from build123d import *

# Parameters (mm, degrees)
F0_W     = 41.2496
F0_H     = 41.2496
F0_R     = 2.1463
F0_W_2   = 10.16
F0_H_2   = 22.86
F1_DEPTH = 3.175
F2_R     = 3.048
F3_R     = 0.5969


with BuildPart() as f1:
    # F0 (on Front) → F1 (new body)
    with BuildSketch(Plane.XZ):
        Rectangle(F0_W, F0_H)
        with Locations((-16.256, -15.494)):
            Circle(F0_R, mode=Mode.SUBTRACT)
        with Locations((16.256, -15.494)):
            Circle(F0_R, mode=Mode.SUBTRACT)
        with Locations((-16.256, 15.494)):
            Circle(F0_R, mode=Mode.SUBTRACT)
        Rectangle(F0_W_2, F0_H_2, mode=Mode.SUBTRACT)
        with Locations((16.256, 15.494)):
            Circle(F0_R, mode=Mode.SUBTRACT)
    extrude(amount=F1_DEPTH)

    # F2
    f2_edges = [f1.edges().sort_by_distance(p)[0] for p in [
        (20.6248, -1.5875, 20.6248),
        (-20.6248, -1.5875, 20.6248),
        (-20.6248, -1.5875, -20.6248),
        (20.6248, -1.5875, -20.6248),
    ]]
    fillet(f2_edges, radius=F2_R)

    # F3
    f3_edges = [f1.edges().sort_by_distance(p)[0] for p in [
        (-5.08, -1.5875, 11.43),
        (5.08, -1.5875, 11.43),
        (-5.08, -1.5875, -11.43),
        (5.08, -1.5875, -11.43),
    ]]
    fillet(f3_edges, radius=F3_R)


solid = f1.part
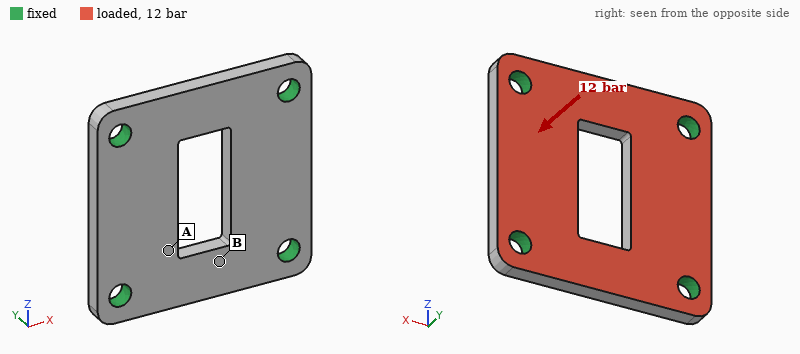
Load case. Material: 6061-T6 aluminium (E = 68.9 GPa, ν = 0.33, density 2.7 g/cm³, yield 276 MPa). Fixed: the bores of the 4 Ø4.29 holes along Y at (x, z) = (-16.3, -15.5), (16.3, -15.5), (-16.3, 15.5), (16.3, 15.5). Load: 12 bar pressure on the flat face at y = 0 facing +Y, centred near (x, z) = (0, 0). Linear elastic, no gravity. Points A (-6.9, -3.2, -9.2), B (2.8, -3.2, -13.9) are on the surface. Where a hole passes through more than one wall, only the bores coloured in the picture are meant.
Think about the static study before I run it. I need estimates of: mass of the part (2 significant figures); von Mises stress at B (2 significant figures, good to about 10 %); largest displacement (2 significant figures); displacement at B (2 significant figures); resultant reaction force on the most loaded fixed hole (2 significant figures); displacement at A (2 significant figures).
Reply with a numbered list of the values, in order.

1. 12 g
2. 28 MPa
3. 33 µm
4. 19 µm
5. 420 N
6. 21 µm
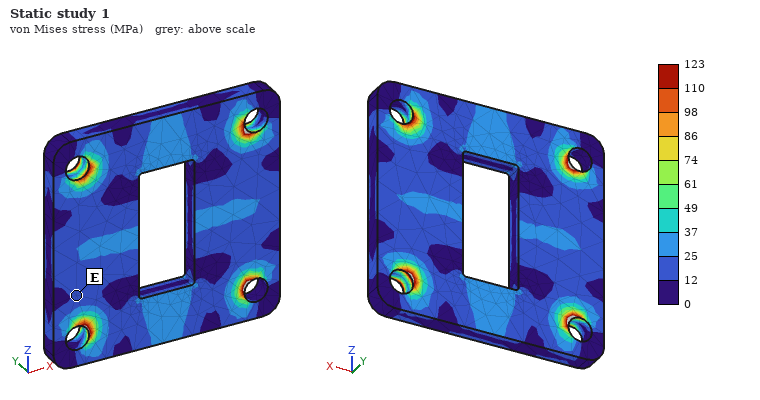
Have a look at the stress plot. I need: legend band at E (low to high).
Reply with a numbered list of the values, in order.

1. 12 to 25 MPa
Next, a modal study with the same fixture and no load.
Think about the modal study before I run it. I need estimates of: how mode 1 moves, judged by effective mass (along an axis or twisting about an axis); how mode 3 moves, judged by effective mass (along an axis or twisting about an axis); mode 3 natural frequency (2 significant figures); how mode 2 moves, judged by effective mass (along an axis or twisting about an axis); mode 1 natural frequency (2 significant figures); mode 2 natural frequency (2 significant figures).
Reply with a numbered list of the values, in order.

1. along Y
2. twisting about X
3. 19 kHz
4. twisting about Z
5. 14 kHz
6. 17 kHz
